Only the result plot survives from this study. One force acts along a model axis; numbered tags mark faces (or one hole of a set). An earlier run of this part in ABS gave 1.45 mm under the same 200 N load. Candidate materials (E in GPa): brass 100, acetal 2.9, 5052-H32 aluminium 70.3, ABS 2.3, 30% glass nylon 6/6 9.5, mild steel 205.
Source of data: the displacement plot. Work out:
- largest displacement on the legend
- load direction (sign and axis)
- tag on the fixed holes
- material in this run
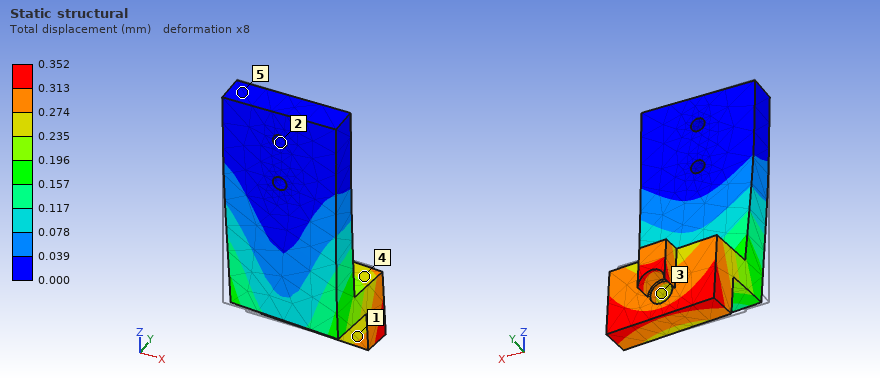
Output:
0.352 mm
+X
2
30% glass nylon 6/6
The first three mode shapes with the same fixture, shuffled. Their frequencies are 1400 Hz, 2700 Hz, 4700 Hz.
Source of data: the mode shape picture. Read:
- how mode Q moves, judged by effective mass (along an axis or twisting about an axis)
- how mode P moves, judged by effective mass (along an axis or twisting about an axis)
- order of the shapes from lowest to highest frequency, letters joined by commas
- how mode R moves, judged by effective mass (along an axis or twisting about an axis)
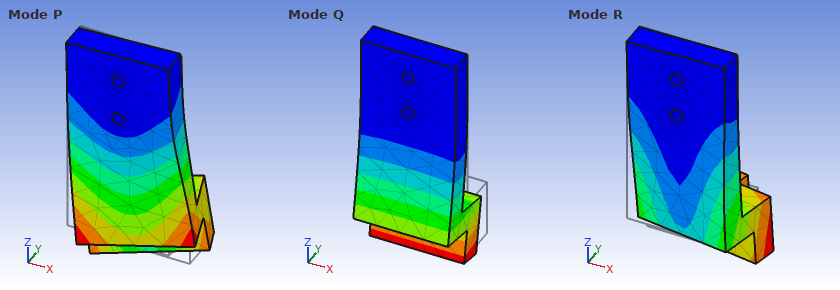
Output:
along Y
along X
Q, R, P
along X
